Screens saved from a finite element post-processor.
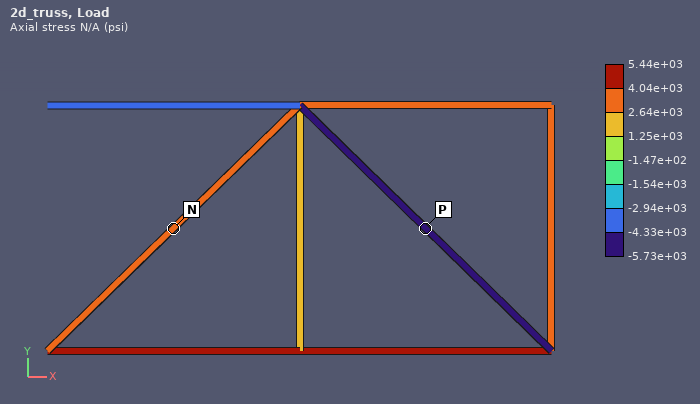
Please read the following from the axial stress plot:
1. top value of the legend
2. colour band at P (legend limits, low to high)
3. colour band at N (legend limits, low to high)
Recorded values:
5.44e+03 psi
-5.73e+03 to -4.33e+03 psi
2.64e+03 to 4.04e+03 psi
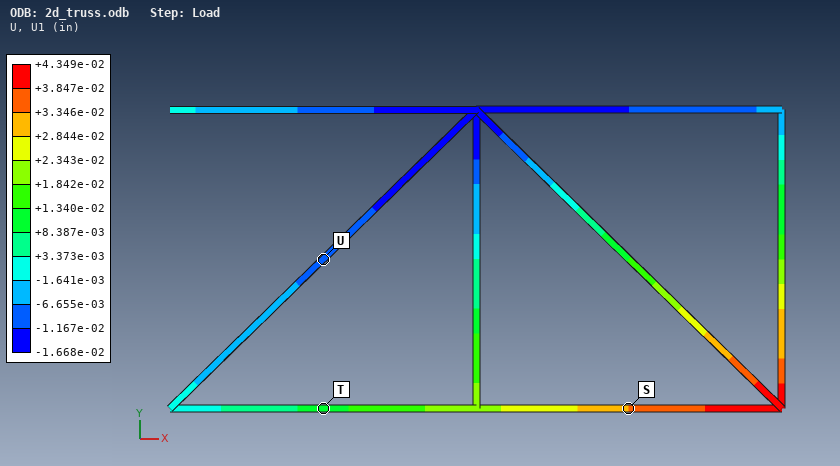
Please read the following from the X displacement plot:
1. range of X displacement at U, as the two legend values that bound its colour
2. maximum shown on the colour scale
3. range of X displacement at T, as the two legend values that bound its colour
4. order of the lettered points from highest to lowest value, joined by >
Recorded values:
-1.167e-02 to -6.655e-03 in
+4.349e-02 in
+8.387e-03 to +1.340e-02 in
S > T > U
